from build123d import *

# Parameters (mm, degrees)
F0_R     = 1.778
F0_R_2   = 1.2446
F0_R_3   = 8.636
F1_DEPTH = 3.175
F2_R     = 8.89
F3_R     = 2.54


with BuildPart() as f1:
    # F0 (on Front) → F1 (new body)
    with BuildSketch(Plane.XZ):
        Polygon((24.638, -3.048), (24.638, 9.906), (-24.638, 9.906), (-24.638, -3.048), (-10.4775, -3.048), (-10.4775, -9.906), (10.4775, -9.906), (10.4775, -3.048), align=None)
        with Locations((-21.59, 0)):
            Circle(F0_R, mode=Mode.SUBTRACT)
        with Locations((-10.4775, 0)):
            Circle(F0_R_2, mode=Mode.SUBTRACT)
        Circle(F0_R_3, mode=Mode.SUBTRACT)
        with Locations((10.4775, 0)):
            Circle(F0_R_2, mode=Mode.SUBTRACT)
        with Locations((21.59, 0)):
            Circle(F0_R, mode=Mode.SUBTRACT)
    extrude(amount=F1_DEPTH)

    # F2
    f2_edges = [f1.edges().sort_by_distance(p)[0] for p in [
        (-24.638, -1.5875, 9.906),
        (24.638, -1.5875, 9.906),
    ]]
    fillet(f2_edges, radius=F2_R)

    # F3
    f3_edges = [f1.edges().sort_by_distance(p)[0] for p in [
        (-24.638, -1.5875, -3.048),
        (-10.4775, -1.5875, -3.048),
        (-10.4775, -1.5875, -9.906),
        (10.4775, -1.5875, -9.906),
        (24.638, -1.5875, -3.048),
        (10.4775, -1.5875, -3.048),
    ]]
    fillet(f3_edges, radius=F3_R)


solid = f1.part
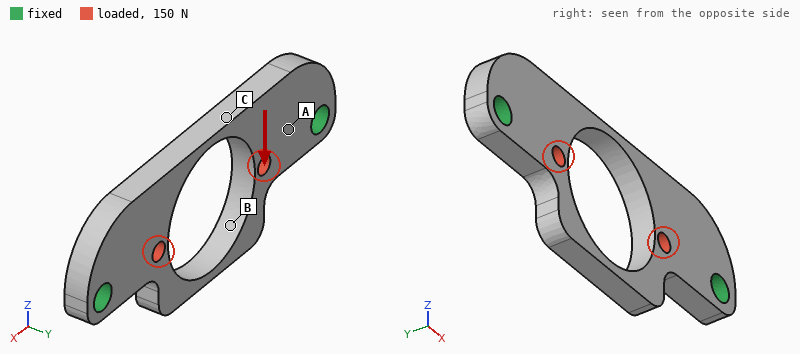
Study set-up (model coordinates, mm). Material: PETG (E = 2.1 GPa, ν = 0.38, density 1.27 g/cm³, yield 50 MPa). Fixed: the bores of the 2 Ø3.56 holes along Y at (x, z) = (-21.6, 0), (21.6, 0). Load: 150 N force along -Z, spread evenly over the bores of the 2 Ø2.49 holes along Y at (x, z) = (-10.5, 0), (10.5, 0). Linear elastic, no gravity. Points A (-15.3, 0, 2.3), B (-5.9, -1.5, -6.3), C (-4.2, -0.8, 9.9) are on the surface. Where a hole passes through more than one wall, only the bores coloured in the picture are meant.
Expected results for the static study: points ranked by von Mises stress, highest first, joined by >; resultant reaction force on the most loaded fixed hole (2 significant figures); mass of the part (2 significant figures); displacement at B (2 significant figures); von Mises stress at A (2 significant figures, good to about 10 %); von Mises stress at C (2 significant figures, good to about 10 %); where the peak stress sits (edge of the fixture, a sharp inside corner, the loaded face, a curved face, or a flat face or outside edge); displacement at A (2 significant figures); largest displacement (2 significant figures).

C > A > B
83 N
1.9 g
82 µm
4.9 MPa
11 MPa
edge of the fixture
46 µm
98 µm
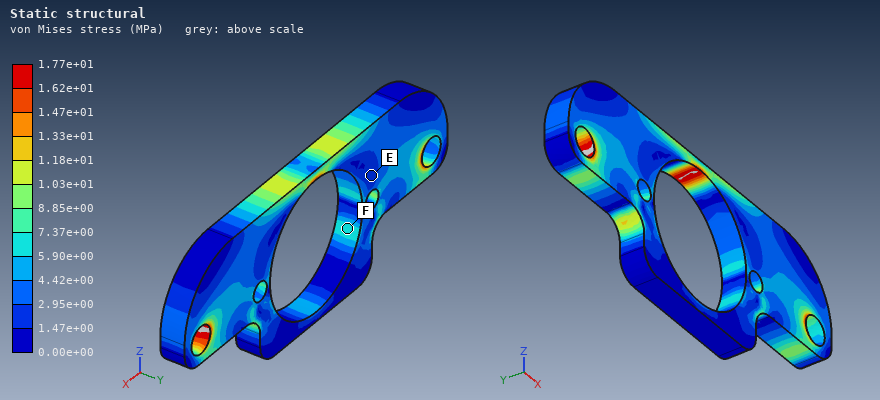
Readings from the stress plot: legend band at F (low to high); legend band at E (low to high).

5.90e+00 to 7.37e+00 MPa
1.47e+00 to 2.95e+00 MPa
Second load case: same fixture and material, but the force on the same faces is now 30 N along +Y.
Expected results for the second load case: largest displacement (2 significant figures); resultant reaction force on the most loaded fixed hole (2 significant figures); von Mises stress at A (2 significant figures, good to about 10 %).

0.16 mm
15 N
2.9 MPa
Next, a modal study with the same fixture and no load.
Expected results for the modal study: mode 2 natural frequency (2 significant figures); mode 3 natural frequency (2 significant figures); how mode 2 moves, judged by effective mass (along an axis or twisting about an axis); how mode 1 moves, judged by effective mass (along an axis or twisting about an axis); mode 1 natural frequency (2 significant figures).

2500 Hz
4400 Hz
along Y
along Y
2100 Hz
